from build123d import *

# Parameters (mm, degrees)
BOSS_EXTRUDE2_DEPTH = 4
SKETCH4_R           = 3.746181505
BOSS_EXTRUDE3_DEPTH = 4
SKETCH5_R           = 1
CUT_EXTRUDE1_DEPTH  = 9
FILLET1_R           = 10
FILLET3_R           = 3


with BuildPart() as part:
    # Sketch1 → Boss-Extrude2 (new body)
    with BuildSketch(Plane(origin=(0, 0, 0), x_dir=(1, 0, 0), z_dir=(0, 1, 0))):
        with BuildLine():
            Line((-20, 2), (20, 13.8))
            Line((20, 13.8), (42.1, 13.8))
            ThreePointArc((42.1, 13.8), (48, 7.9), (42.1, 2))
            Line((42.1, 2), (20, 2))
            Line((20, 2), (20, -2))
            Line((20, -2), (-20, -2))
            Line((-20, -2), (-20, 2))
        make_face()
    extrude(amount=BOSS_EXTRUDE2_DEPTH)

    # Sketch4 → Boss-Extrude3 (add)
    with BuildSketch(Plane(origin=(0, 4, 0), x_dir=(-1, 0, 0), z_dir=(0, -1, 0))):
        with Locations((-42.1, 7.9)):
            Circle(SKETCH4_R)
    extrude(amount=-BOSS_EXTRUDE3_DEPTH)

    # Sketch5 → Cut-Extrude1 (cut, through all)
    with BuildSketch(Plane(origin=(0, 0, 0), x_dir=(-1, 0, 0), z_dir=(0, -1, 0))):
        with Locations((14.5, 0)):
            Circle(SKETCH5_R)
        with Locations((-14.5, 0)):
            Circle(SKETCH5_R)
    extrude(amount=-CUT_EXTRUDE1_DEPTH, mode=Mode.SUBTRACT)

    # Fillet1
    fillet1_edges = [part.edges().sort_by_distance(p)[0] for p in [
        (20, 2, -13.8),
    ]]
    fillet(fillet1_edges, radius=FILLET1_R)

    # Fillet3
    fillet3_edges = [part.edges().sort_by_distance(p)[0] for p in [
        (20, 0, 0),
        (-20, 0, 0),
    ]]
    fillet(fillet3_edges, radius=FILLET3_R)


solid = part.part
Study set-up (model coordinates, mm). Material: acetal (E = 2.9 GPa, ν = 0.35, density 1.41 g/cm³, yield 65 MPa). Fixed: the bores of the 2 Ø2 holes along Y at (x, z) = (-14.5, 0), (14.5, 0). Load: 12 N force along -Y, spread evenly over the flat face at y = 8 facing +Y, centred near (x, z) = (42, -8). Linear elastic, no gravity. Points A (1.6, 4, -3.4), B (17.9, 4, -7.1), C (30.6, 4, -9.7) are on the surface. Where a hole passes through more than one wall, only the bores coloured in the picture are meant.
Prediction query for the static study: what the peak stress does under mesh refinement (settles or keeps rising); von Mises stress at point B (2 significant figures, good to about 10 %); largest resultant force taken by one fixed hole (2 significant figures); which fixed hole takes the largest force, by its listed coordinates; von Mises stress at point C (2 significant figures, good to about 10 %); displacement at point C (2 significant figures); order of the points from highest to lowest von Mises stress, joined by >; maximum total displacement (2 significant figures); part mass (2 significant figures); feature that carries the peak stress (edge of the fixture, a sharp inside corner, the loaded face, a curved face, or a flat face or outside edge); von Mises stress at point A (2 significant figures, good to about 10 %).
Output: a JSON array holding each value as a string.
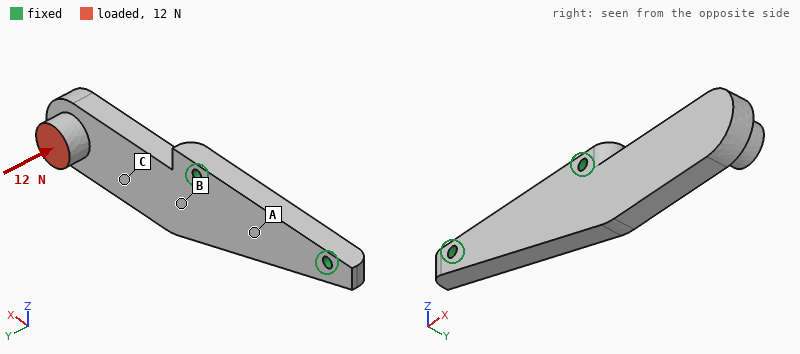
["keeps rising", "8.3 MPa", "17 N", "(14.5, 0)", "4.4 MPa", "0.31 mm", "B > C > A", "0.81 mm", "4.2 g", "edge of the fixture", "1.6 MPa"]
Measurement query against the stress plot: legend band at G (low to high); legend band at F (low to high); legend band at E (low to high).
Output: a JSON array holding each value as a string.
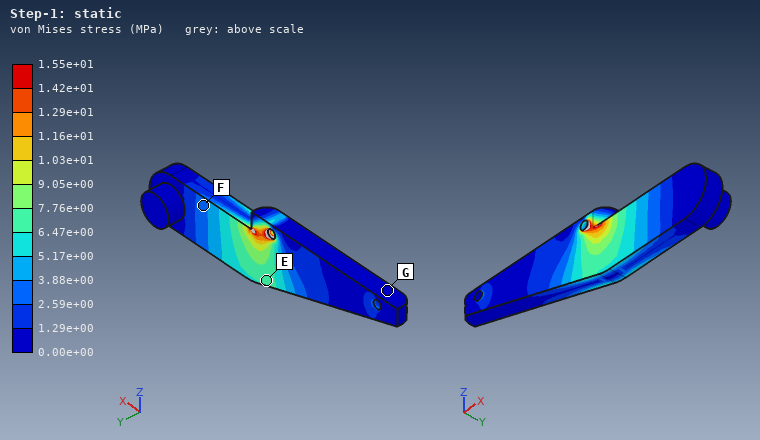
["0.00e+00 to 1.29e+00 MPa", "2.59e+00 to 3.88e+00 MPa", "6.47e+00 to 7.76e+00 MPa"]
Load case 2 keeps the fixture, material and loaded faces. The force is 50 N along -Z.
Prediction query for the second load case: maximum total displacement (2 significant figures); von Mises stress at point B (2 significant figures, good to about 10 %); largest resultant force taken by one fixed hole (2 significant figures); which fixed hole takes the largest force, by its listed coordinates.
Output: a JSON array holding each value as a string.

["0.75 mm", "9.7 MPa", "120 N", "(14.5, 0)"]
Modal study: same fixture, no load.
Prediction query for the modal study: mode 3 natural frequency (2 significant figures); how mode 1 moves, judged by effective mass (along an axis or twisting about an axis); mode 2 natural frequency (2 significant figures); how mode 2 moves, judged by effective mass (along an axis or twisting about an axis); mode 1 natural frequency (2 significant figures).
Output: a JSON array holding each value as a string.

["2600 Hz", "along Y", "1600 Hz", "along Z", "650 Hz"]
